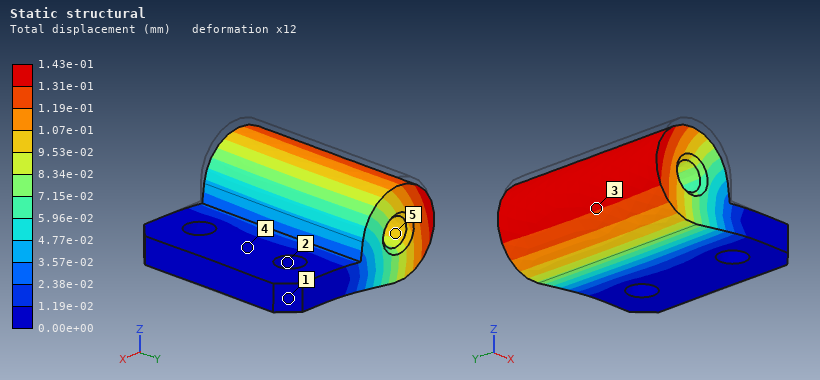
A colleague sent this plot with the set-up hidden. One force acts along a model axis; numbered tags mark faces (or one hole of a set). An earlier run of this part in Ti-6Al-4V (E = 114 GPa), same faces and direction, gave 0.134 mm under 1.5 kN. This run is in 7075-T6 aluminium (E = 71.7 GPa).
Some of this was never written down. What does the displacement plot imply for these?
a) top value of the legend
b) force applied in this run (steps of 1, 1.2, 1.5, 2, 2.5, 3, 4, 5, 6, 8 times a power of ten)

1.43e-01 mm
1 kN
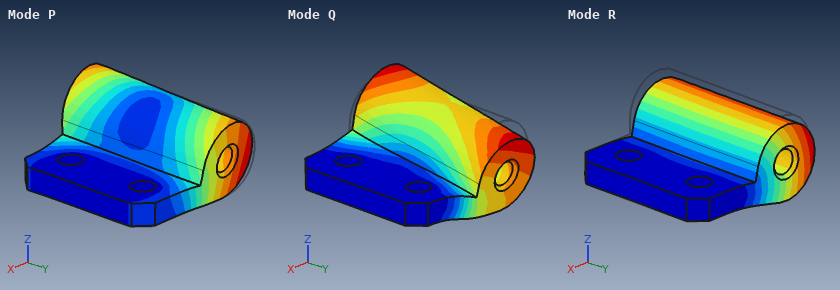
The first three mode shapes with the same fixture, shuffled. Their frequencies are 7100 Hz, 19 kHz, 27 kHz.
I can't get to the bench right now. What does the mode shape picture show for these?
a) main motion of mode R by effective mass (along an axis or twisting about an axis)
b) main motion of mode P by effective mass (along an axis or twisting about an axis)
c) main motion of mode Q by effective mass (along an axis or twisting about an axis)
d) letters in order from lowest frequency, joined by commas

along Z
along Y
along Y
R, Q, P
